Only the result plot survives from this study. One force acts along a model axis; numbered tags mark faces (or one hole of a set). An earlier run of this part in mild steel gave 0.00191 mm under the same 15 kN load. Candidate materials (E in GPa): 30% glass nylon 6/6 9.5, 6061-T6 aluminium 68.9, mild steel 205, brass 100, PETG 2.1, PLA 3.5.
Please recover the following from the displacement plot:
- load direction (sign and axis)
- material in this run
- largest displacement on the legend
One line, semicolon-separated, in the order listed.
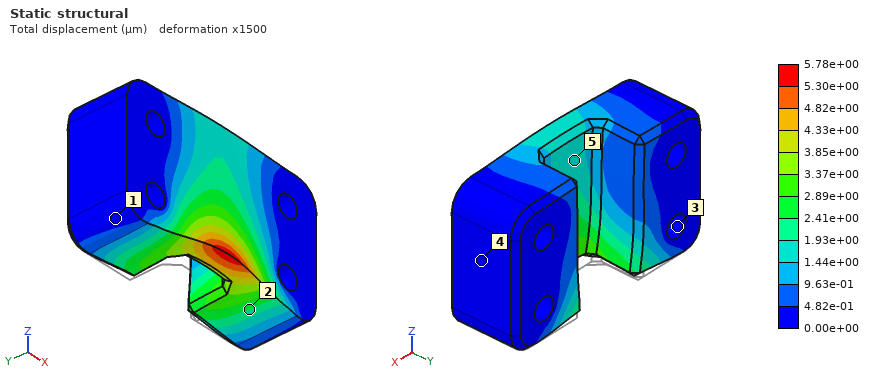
+Z; 6061-T6 aluminium; 5.78e+00 µm
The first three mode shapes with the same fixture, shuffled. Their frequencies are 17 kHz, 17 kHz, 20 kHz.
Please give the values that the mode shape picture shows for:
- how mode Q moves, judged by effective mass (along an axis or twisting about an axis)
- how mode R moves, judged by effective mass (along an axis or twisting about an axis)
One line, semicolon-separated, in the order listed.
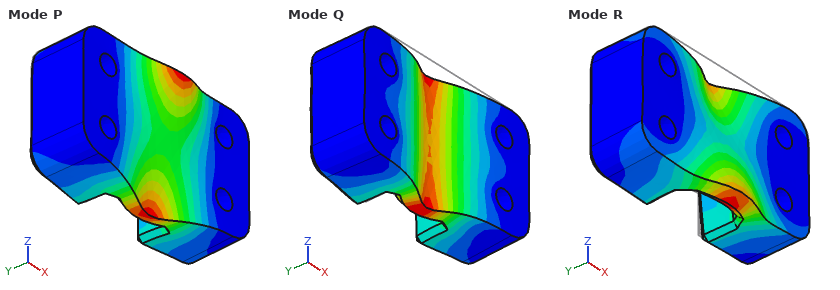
along Y; along Z
